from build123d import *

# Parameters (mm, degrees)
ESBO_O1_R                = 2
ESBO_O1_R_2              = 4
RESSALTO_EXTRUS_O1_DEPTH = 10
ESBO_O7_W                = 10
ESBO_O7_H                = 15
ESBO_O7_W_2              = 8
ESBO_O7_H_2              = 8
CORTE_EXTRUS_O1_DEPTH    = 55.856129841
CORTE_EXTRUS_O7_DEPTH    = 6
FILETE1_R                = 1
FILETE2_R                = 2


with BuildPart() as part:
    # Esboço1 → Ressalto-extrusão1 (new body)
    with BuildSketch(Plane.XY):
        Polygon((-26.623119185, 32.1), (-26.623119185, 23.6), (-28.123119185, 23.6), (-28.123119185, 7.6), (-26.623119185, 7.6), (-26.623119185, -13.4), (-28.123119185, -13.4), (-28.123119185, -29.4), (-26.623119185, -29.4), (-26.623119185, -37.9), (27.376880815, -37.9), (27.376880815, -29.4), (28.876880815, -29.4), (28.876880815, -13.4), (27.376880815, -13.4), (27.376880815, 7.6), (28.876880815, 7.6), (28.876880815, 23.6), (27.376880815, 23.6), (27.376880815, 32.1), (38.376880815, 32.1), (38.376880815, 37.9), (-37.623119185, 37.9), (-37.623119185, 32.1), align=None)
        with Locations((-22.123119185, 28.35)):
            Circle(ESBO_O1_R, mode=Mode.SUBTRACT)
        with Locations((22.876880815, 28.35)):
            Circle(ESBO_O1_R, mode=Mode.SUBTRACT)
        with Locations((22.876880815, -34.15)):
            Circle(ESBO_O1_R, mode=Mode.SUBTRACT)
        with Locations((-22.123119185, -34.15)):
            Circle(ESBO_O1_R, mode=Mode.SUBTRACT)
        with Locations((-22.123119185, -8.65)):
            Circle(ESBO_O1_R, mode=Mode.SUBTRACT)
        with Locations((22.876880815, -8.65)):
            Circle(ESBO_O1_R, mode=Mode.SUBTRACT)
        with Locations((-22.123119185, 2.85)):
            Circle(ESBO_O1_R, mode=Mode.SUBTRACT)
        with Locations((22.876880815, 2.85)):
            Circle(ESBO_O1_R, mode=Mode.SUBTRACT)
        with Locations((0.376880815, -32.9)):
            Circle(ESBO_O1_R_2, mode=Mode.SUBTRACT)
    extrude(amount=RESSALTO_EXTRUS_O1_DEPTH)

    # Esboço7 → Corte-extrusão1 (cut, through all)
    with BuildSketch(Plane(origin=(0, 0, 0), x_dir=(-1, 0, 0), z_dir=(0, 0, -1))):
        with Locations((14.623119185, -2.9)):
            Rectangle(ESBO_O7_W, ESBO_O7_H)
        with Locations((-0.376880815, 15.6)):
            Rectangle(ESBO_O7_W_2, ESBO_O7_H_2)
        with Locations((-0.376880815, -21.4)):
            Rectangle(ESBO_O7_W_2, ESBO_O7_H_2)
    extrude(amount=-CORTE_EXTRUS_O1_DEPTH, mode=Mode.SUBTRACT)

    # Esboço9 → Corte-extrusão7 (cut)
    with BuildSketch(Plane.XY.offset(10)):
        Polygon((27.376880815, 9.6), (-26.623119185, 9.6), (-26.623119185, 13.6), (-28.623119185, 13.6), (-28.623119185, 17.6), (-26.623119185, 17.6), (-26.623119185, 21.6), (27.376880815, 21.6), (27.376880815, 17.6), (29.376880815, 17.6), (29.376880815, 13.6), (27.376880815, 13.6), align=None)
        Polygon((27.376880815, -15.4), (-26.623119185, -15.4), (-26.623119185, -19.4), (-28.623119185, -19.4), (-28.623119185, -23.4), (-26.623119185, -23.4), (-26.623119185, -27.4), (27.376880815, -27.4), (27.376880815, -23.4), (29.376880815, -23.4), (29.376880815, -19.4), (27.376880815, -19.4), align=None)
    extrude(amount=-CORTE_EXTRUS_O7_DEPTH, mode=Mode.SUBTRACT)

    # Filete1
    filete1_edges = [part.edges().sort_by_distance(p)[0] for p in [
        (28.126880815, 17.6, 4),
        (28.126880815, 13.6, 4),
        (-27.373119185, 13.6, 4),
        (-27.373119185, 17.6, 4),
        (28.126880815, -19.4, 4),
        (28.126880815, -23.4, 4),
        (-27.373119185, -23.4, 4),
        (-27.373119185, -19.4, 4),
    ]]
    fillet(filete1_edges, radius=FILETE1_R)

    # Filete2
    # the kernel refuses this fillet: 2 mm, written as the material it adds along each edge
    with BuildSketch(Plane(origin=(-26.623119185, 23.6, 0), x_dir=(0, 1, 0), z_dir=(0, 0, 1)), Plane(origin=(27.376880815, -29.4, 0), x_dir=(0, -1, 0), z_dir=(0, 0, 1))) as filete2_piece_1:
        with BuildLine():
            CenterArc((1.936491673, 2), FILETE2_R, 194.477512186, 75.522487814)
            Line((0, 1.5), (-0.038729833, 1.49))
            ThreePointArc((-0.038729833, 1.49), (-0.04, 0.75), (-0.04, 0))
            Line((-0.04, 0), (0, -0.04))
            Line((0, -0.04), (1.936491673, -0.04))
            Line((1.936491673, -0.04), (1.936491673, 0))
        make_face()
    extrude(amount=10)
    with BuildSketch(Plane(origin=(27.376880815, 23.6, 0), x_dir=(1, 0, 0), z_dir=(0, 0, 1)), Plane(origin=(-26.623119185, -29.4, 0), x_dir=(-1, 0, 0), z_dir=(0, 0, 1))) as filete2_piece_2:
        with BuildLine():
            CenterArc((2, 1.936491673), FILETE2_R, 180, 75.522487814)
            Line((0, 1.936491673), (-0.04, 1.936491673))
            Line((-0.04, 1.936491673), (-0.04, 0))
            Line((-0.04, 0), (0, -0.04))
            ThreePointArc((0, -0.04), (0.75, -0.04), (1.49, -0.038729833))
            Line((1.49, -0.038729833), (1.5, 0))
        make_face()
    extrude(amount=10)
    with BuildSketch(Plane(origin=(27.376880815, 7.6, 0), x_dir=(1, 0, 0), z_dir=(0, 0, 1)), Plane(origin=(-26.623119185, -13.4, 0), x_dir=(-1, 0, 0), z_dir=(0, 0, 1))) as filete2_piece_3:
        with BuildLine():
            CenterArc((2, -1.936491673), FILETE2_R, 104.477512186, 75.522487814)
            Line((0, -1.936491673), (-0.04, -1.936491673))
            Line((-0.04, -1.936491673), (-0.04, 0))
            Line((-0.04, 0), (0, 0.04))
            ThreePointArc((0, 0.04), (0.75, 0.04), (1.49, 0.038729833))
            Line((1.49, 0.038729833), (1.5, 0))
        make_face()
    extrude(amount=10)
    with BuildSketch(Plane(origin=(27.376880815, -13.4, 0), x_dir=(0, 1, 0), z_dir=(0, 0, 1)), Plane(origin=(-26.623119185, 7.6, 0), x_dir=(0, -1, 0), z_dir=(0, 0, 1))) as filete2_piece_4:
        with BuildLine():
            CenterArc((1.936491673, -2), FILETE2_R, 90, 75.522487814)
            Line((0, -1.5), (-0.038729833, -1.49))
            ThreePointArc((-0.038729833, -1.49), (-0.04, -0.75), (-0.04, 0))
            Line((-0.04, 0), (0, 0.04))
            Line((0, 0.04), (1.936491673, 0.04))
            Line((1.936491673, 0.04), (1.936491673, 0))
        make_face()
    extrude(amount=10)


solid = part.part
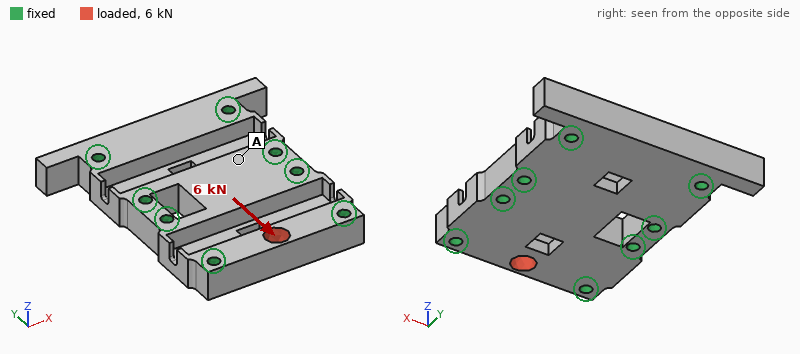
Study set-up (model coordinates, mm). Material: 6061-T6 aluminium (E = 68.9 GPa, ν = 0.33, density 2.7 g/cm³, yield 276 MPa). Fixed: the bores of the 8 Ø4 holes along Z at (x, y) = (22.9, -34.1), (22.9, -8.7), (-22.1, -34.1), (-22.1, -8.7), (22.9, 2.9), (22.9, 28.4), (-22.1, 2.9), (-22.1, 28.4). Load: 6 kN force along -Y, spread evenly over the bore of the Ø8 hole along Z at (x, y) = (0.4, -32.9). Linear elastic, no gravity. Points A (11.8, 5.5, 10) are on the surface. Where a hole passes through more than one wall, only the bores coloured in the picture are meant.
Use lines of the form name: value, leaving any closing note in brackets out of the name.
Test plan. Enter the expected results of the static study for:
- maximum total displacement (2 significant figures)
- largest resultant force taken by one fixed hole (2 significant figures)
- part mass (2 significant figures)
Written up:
maximum total displacement: 49 µm
largest resultant force taken by one fixed hole: 1.8 kN
part mass: 86 g
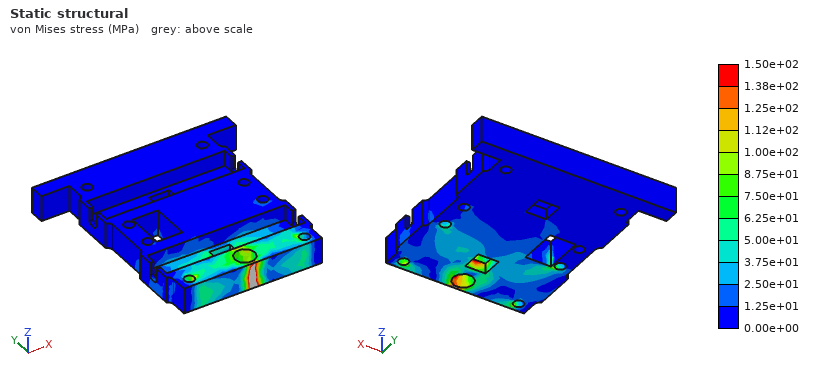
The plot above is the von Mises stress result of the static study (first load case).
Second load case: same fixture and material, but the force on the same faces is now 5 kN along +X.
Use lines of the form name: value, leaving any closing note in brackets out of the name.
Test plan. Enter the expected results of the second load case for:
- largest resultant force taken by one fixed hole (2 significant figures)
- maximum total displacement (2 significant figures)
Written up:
largest resultant force taken by one fixed hole: 2.2 kN
maximum total displacement: 8.3 µm
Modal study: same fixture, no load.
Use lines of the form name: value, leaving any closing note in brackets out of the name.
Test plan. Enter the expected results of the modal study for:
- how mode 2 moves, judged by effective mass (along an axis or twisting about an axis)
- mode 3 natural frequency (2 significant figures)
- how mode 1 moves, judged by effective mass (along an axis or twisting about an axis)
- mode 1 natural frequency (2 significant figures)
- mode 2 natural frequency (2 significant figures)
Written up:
how mode 2 moves, judged by effective mass: twisting about X
mode 3 natural frequency: 20 kHz
how mode 1 moves, judged by effective mass: along Z
mode 1 natural frequency: 17 kHz
mode 2 natural frequency: 19 kHz
